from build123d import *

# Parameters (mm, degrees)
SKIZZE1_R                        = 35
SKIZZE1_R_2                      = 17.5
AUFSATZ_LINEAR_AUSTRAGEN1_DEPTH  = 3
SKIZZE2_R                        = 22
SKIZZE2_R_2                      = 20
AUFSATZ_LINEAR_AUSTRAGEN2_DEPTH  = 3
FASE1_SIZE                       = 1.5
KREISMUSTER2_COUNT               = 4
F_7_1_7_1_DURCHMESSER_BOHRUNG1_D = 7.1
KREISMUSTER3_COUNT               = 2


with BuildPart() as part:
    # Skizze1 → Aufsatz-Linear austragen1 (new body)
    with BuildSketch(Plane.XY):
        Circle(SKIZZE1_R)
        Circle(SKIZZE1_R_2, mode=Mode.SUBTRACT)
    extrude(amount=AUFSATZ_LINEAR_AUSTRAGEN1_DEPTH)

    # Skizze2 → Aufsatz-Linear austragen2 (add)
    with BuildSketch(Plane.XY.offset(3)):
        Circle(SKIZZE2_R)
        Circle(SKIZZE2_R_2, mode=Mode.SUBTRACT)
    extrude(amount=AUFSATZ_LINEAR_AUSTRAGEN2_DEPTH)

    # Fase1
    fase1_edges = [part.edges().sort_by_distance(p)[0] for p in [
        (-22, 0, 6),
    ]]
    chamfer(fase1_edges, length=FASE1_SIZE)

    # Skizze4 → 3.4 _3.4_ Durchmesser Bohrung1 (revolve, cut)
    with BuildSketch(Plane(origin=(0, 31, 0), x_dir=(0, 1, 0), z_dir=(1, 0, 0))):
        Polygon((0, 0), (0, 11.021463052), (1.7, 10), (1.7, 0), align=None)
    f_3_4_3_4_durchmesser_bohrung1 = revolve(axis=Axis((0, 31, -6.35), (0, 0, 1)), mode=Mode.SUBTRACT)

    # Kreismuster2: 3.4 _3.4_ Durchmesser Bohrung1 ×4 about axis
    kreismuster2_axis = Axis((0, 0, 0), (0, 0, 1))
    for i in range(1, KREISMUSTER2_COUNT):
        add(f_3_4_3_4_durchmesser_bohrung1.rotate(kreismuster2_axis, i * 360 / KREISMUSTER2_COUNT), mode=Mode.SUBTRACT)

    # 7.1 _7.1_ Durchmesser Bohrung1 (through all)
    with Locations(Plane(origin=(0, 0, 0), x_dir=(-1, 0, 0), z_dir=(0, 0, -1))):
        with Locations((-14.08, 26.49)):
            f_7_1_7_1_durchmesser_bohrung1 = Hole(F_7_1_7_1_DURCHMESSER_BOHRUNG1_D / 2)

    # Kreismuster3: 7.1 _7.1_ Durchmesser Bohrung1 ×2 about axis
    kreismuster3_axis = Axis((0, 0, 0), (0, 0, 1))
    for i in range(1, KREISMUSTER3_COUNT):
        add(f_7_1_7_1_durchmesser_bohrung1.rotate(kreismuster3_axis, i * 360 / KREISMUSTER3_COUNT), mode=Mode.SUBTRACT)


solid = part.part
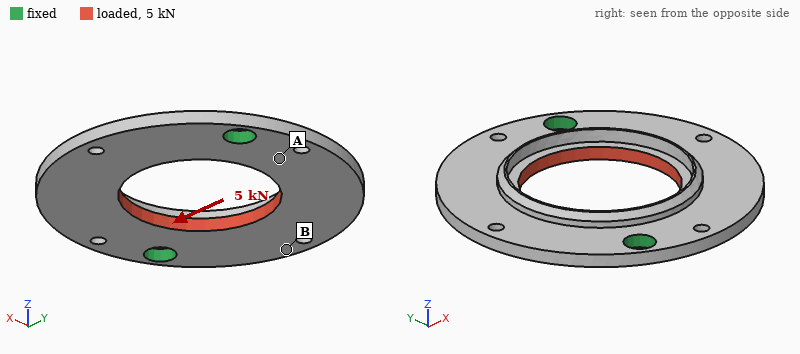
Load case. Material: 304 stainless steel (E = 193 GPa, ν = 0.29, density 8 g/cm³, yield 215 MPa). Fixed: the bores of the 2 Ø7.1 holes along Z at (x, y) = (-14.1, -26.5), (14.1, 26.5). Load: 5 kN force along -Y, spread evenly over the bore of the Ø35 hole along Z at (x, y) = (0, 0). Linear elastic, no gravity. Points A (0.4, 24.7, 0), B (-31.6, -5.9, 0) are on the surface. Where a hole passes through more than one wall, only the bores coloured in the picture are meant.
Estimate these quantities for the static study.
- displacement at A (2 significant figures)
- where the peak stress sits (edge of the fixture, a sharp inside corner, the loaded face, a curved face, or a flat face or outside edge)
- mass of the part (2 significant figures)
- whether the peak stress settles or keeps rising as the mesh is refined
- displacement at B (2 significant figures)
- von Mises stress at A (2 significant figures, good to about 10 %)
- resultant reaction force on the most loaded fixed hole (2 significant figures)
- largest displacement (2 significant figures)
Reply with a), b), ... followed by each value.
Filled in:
a) 4.6 µm
b) edge of the fixture
c) 72 g
d) keeps rising
e) 5.0 µm
f) 30 MPa
g) 2.5 kN
h) 8.1 µm
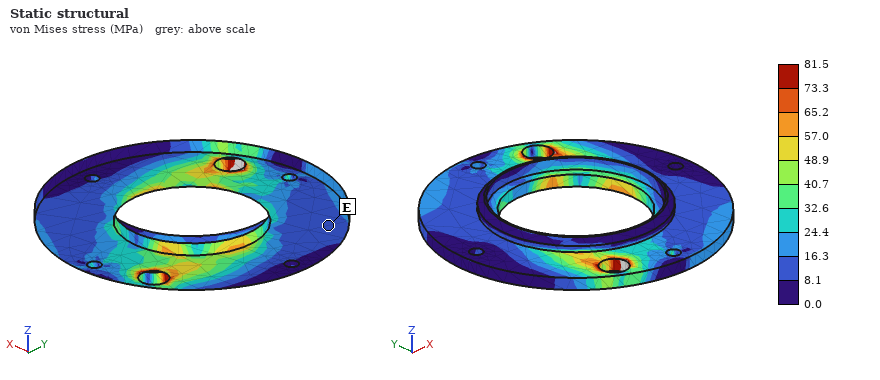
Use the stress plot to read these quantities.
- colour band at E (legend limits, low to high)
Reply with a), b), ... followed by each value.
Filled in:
a) 8.1 to 16.3 MPa
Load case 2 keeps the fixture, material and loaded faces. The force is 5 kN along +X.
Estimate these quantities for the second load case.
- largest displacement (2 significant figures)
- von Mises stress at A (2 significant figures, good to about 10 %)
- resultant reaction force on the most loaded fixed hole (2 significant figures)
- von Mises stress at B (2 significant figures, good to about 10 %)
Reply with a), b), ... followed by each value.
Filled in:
a) 8.1 µm
b) 40 MPa
c) 2.5 kN
d) 18 MPa
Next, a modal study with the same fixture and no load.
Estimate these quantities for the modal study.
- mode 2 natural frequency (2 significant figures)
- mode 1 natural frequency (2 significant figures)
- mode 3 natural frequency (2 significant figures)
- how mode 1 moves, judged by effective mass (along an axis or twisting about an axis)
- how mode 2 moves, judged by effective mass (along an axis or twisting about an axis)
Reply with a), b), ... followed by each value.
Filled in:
a) 2300 Hz
b) 1900 Hz
c) 5500 Hz
d) twisting about Y
e) along Z
